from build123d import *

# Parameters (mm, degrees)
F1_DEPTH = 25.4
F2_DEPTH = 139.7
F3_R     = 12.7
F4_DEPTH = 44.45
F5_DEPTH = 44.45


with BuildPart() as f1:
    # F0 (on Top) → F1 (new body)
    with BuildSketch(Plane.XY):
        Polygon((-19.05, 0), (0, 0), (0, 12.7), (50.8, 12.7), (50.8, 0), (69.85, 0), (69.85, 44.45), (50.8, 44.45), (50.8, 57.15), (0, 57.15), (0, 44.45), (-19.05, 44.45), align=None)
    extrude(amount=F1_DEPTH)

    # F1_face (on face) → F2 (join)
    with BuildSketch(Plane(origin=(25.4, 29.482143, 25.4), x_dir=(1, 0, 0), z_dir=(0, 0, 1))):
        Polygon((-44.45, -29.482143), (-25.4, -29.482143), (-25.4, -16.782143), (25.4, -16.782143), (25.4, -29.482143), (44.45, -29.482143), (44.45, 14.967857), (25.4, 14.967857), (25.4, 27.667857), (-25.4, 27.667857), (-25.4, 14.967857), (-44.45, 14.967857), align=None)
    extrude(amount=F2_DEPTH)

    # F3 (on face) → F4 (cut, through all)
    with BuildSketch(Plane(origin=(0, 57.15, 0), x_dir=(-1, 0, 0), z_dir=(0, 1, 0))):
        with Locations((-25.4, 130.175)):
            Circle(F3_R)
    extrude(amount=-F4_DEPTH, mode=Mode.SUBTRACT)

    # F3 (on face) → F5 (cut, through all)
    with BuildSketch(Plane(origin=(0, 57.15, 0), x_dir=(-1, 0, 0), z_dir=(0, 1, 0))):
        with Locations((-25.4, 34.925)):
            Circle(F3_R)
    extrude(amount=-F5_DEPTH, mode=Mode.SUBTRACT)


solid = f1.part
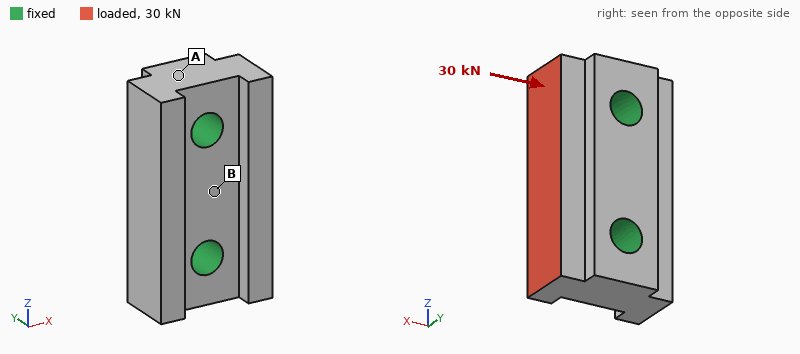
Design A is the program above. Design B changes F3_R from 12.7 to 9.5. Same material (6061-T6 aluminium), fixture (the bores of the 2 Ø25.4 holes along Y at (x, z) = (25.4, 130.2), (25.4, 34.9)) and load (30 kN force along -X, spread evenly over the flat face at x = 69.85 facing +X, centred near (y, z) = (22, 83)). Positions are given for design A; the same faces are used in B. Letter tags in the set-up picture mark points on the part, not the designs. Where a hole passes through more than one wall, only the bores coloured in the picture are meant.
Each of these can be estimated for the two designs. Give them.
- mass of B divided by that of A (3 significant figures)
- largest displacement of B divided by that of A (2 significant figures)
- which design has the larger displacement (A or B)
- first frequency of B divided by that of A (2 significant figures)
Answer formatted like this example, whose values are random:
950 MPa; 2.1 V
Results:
1.03; 1.1; B; 0.87
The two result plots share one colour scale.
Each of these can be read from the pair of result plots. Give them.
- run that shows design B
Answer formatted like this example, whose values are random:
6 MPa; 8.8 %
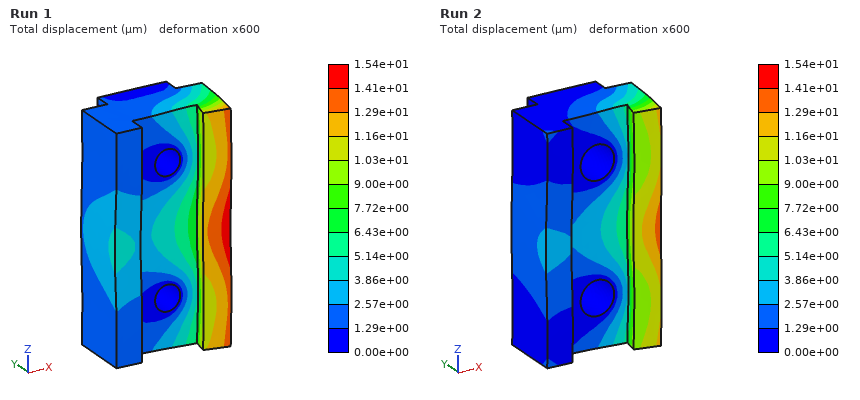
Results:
Run 1
